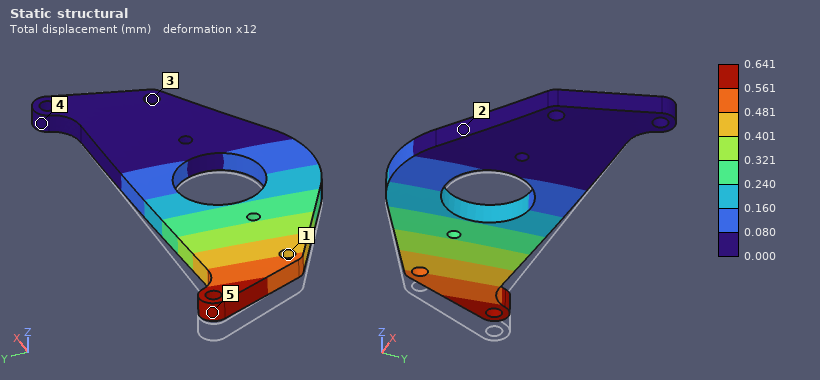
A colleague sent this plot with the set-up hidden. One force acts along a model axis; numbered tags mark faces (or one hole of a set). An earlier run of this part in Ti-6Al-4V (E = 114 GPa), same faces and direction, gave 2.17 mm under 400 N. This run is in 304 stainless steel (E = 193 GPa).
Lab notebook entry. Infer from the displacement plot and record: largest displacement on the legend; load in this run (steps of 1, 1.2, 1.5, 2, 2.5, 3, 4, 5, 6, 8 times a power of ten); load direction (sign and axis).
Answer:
0.641 mm
200 N
+Z
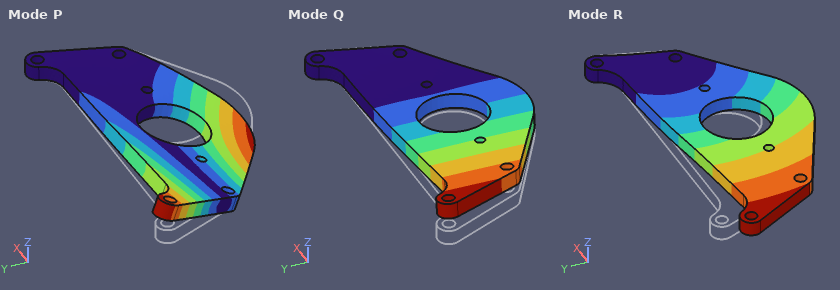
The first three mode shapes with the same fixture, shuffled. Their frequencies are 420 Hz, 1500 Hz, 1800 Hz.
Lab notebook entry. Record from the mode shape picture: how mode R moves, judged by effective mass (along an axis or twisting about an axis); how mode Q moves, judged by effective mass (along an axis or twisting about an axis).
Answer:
along Y
along Z
